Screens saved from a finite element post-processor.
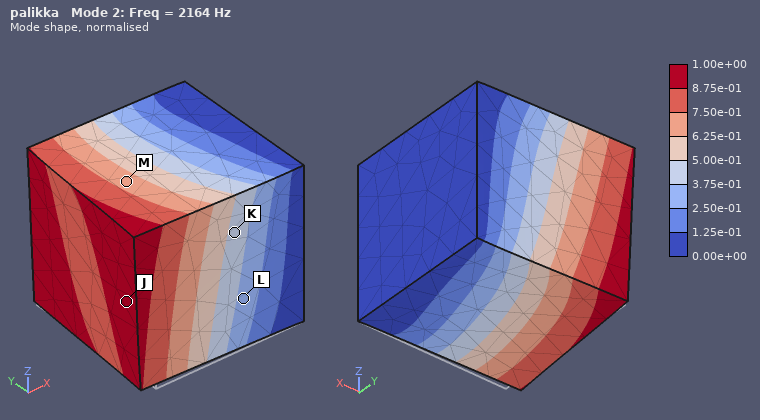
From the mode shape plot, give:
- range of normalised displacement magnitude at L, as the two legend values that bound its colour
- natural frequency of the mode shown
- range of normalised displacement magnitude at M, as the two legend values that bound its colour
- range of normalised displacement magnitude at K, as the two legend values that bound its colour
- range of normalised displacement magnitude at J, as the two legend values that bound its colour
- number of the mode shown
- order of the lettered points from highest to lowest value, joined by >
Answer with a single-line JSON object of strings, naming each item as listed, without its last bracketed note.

{"range of normalised displacement magnitude at L, as the two legend values that bound its colour": "2.50e-01 to 3.75e-01", "natural frequency of the mode shown": "2164 Hz", "range of normalised displacement magnitude at M, as the two legend values that bound its colour": "6.25e-01 to 7.50e-01", "range of normalised displacement magnitude at K, as the two legend values that bound its colour": "3.75e-01 to 5.00e-01", "range of normalised displacement magnitude at J, as the two legend values that bound its colour": "8.75e-01 to 1.00e+00", "number of the mode shown": "2", "order of the lettered points from highest to lowest value, joined by >": "J > M > K > L"}
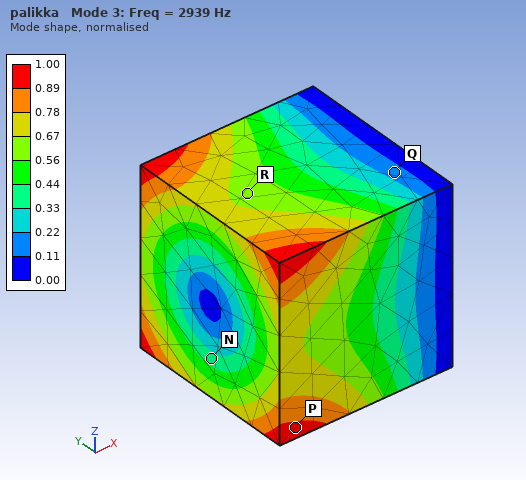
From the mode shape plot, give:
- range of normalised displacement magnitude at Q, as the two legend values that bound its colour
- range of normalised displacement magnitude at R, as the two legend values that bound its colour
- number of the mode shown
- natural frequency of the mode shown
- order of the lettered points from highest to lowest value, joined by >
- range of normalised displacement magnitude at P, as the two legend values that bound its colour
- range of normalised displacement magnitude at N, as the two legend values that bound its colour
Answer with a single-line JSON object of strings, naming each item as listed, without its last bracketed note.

{"range of normalised displacement magnitude at Q, as the two legend values that bound its colour": "0.11 to 0.22", "range of normalised displacement magnitude at R, as the two legend values that bound its colour": "0.56 to 0.67", "number of the mode shown": "3", "natural frequency of the mode shown": "2939 Hz", "order of the lettered points from highest to lowest value, joined by >": "P > R > N > Q", "range of normalised displacement magnitude at P, as the two legend values that bound its colour": "0.89 to 1.00", "range of normalised displacement magnitude at N, as the two legend values that bound its colour": "0.33 to 0.44"}
